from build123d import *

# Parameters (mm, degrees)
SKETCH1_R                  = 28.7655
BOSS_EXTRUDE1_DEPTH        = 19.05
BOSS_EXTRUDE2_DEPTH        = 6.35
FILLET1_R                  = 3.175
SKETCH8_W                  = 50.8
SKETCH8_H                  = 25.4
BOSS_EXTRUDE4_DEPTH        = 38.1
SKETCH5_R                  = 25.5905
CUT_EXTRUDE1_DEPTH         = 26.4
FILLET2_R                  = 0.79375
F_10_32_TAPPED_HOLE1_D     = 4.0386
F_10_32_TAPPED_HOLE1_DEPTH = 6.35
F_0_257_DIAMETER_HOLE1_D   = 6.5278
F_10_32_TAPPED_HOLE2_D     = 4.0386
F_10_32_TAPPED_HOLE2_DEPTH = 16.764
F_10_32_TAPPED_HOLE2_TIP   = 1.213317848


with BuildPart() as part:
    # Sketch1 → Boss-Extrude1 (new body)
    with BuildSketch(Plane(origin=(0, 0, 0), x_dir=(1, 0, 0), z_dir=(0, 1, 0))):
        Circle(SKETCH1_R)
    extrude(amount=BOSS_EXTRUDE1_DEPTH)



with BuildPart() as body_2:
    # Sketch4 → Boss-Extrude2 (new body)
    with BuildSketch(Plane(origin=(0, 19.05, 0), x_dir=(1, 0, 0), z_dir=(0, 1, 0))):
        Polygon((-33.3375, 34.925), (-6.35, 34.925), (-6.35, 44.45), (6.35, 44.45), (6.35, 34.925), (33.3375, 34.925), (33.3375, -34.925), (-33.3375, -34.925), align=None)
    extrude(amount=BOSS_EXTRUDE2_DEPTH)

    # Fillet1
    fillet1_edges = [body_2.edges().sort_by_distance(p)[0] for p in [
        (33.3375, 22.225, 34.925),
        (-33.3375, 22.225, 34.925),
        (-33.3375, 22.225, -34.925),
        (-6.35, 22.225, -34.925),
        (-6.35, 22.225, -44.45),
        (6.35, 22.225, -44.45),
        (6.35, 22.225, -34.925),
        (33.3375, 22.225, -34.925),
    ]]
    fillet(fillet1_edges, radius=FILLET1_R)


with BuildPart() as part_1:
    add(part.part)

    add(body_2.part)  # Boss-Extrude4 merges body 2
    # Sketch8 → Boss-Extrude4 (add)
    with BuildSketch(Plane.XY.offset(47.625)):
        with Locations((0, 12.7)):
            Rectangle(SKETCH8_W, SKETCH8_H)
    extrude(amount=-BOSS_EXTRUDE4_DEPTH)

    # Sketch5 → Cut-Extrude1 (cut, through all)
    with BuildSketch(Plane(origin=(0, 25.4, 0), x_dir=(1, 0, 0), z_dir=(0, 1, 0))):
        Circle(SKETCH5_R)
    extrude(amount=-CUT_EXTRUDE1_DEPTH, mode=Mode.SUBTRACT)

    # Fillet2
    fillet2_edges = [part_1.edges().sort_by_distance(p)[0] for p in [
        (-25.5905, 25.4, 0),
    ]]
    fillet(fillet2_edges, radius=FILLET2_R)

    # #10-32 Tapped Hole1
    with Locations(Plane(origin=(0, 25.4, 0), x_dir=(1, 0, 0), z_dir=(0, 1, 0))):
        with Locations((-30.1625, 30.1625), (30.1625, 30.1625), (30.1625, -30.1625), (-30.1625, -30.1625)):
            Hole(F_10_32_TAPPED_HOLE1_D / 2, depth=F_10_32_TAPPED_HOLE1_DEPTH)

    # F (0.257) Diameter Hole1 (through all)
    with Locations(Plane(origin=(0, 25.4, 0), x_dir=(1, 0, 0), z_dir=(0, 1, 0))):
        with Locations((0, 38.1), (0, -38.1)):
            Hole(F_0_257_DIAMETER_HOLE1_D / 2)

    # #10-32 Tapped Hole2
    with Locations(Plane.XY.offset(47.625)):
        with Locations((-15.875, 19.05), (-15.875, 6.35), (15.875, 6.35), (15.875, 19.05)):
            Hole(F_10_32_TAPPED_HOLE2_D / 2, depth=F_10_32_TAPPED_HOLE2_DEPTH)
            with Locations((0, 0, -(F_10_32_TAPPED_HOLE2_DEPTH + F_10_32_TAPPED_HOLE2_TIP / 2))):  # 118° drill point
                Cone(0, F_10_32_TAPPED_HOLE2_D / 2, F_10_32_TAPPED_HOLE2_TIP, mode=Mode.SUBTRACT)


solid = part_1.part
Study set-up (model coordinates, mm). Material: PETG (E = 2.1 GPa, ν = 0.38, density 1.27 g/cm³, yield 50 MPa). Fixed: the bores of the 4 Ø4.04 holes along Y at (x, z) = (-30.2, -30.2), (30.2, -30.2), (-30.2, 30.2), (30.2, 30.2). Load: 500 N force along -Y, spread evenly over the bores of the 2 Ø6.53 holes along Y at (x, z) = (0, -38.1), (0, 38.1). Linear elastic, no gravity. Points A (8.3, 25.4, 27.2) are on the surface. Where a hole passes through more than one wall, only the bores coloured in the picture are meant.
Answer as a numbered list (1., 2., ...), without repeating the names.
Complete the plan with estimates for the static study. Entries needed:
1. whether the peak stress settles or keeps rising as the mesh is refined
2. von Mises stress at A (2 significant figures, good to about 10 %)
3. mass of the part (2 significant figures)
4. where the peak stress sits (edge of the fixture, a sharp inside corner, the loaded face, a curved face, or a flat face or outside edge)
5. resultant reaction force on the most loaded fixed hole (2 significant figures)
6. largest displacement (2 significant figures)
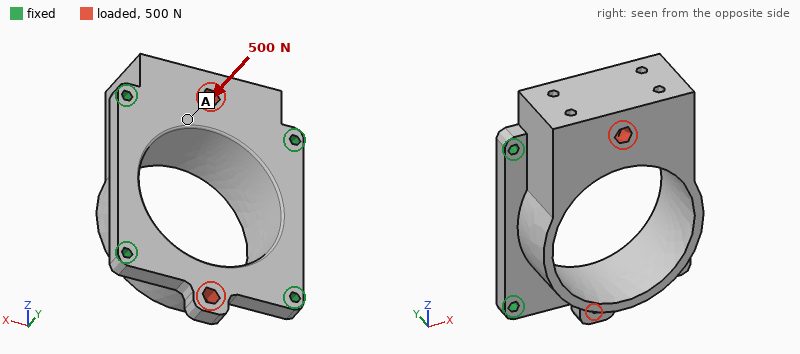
1. keeps rising
2. 1.0 MPa
3. 66 g
4. edge of the fixture
5. 260 N
6. 0.41 mm
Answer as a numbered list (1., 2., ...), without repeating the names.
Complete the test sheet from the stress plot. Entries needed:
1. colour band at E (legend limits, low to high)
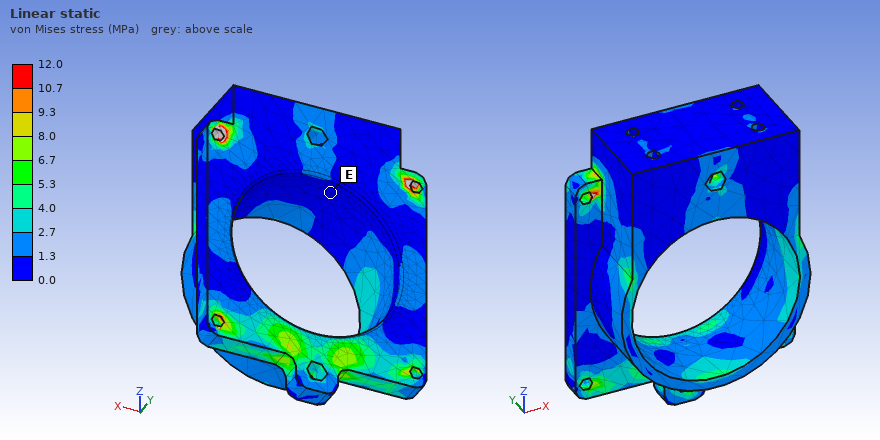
1. 0.0 to 1.3 MPa
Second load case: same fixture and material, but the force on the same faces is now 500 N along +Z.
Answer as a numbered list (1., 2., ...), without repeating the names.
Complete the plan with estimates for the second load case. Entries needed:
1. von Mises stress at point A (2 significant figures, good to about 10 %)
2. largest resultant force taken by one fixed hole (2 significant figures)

1. 0.63 MPa
2. 160 N
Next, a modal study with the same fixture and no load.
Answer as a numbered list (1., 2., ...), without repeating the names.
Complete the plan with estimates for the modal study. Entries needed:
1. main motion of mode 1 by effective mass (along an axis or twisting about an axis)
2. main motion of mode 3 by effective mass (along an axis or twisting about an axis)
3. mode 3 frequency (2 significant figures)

1. along Z
2. along Y
3. 2200 Hz
